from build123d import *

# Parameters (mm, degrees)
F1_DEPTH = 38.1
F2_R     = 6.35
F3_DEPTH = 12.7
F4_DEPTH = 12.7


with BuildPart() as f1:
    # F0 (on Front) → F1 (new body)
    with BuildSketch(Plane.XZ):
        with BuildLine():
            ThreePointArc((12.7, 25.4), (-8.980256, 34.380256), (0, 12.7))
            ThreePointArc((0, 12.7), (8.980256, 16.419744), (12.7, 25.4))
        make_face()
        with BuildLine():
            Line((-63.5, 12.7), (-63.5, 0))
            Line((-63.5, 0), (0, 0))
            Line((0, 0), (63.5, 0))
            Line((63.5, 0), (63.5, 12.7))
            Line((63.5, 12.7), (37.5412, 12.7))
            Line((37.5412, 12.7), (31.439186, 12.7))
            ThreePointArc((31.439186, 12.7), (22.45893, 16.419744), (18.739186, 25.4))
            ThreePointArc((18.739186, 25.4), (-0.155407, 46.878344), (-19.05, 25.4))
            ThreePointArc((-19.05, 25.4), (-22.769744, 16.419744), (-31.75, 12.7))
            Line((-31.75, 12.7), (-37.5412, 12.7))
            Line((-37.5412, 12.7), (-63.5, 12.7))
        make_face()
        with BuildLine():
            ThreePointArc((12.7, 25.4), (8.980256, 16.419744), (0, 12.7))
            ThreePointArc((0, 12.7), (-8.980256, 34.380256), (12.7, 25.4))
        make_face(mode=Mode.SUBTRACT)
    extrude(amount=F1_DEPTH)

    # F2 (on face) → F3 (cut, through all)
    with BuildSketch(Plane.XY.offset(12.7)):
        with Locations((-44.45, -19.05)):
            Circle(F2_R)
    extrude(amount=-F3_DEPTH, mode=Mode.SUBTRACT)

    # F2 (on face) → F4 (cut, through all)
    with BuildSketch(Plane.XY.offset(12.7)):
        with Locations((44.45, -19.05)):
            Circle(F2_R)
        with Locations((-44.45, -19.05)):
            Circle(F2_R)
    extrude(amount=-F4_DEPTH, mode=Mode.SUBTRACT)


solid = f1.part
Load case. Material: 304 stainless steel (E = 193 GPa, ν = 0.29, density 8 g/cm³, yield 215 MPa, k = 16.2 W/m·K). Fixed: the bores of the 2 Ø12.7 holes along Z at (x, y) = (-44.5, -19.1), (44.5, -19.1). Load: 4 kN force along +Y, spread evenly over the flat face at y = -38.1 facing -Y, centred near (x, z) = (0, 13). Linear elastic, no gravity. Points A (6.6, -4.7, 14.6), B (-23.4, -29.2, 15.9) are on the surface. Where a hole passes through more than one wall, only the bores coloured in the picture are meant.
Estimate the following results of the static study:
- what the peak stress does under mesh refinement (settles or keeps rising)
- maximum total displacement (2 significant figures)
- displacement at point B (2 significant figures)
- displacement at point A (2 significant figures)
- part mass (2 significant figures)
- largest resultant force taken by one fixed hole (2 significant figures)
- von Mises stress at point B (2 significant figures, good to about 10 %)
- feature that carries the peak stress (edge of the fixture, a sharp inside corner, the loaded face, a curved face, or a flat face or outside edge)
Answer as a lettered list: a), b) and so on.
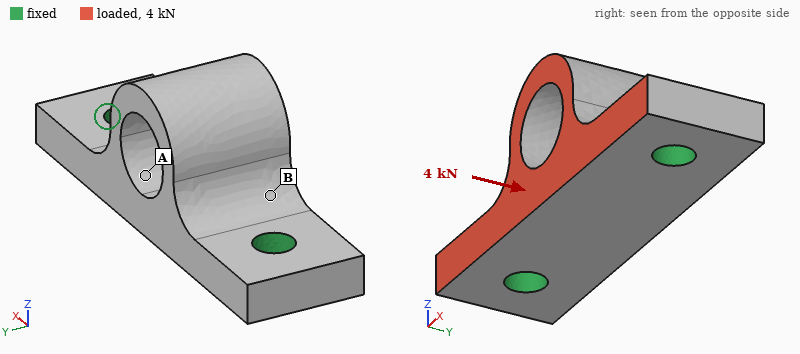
a) keeps rising
b) 9.0 µm
c) 2.9 µm
d) 3.6 µm
e) 680 g
f) 2.0 kN
g) 11 MPa
h) edge of the fixture
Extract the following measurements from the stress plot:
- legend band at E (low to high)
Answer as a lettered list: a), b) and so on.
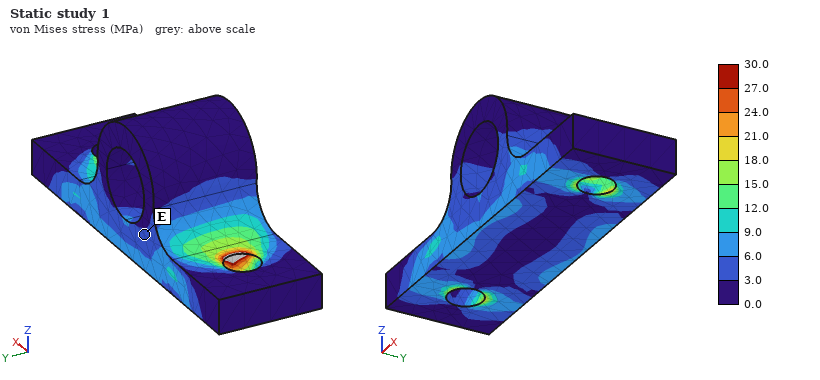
a) 3.0 to 6.0 MPa
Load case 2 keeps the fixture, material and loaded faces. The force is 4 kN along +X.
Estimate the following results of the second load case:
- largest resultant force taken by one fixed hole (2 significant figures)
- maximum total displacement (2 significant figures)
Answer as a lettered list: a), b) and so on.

a) 2.2 kN
b) 4.2 µm
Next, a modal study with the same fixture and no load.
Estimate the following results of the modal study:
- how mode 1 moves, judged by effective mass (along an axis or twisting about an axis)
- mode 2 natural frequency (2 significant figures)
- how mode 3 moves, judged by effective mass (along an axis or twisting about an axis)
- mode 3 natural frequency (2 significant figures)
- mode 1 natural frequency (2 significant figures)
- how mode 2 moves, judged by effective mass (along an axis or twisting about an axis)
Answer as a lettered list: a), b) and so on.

a) along Y
b) 7000 Hz
c) along X
d) 9000 Hz
e) 4600 Hz
f) along Z
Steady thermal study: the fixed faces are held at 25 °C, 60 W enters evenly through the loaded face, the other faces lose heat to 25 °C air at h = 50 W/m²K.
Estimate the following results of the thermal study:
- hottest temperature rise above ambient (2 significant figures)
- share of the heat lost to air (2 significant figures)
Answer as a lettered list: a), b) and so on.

a) 60 K
b) 36 %
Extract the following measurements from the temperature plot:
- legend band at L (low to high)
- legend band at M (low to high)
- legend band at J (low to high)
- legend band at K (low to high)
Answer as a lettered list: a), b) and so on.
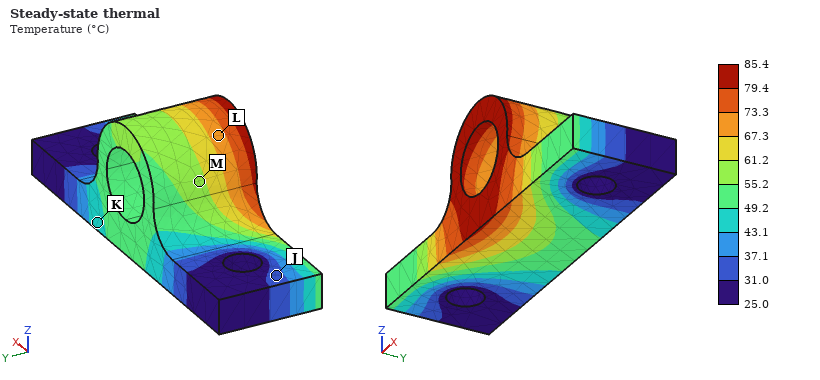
a) 67.3 to 73.3 °C
b) 55.2 to 61.2 °C
c) 31.0 to 37.1 °C
d) 43.1 to 49.2 °C
